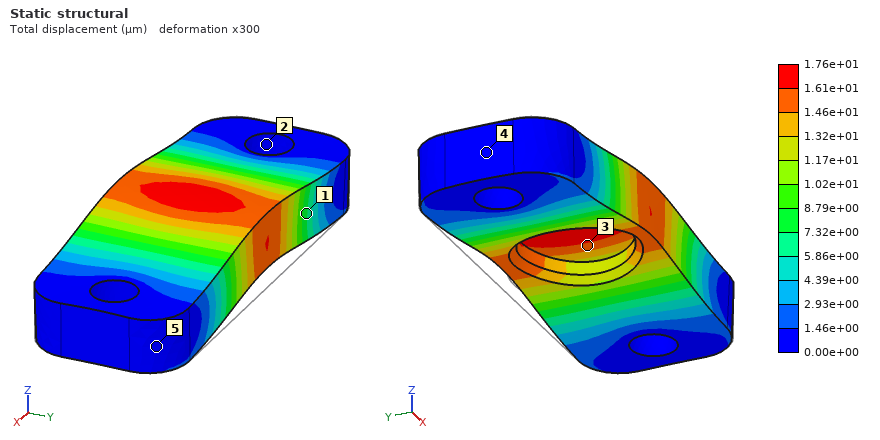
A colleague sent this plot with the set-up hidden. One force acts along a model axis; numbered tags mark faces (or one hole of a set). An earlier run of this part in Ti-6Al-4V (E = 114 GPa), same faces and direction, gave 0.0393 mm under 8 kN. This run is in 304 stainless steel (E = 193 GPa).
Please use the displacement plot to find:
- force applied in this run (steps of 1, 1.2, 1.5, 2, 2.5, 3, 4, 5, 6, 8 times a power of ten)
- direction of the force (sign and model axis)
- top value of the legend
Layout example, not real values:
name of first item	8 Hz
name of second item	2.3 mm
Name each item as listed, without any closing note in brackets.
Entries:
force applied in this run	6 kN
direction of the force	+Z
top value of the legend	1.76e+01 µm
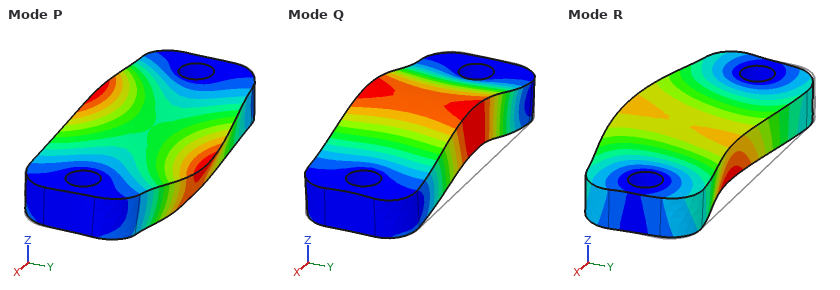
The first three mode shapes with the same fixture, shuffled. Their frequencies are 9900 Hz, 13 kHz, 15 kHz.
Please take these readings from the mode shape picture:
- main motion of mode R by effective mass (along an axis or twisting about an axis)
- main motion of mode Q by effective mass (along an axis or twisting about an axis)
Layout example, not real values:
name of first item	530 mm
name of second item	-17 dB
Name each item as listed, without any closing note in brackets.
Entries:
main motion of mode R by effective mass	along Y
main motion of mode Q by effective mass	along Z
